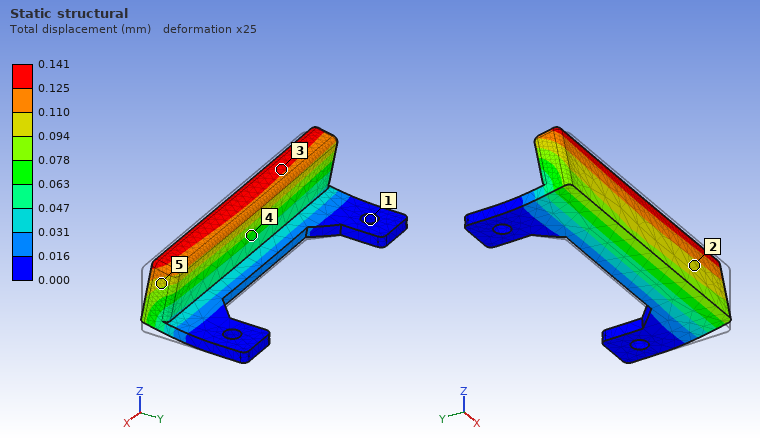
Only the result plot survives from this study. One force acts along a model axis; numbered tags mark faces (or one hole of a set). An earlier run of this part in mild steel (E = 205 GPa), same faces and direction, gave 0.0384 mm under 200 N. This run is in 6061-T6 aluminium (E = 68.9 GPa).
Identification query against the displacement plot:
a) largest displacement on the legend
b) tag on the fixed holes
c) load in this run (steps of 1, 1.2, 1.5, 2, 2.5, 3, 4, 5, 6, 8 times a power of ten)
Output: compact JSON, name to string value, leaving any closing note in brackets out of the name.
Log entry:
{"largest displacement on the legend": "0.141 mm", "tag on the fixed holes": "1", "load in this run": "250 N"}
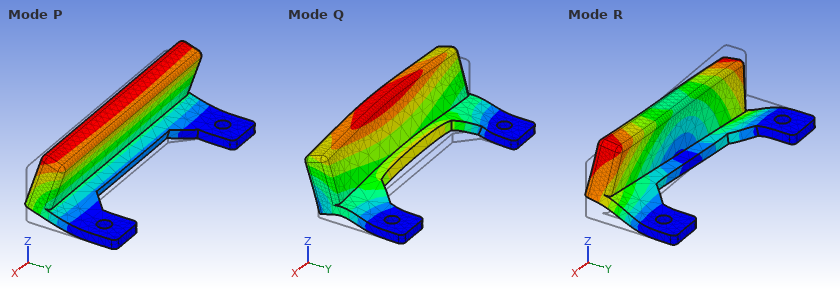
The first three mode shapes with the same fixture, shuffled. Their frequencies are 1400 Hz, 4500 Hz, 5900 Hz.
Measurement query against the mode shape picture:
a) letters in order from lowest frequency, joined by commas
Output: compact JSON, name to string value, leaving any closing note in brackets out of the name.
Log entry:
{"letters in order from lowest frequency, joined by commas": "P, R, Q"}
